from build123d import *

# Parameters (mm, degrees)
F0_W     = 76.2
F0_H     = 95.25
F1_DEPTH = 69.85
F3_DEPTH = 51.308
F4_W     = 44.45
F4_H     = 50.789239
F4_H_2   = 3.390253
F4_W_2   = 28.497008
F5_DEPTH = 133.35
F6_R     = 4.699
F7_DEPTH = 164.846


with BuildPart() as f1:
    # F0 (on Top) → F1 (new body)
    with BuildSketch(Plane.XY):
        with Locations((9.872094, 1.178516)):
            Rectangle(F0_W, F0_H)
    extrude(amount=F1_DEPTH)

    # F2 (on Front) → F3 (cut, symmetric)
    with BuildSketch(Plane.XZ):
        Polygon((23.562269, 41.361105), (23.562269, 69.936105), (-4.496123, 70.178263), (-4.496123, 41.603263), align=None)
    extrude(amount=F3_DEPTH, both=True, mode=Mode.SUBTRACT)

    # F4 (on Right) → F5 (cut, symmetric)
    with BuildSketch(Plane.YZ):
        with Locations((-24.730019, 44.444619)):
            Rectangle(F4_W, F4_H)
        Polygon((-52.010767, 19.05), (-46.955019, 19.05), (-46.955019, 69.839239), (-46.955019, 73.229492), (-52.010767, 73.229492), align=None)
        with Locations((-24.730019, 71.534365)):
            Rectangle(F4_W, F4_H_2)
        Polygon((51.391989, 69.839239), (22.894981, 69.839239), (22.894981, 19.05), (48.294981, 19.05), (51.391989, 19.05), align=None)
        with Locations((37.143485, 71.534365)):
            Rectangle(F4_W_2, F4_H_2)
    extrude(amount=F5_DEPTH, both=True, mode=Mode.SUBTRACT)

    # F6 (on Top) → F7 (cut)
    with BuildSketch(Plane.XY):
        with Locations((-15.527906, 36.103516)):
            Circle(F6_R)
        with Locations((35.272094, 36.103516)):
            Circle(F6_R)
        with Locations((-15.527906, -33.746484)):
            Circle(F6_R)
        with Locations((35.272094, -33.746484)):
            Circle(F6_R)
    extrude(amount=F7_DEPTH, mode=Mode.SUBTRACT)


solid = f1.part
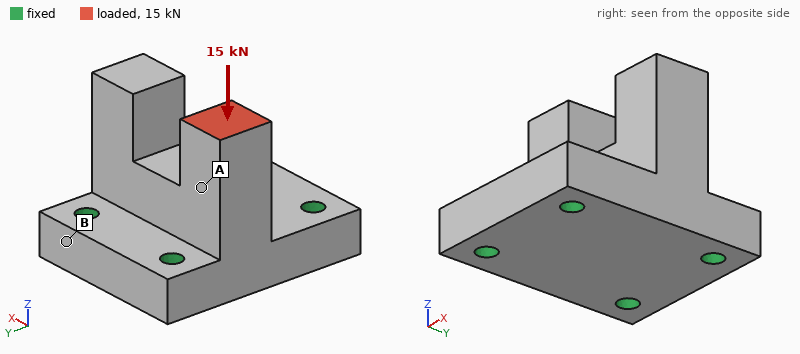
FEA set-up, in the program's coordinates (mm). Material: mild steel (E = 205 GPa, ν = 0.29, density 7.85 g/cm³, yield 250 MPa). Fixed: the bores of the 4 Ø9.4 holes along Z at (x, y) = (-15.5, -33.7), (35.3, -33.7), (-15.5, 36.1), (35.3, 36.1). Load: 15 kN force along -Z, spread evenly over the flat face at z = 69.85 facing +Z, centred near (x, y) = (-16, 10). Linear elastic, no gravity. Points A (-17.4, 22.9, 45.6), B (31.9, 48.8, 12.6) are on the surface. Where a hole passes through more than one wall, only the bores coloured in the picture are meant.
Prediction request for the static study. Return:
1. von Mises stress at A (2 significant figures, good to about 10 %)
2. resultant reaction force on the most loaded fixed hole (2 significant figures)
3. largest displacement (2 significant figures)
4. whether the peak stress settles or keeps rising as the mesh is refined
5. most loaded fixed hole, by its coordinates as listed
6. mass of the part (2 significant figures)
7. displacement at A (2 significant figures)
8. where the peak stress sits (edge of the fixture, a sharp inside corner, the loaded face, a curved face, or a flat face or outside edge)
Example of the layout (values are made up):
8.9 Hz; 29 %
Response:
23 MPa; 9.7 kN; 21 µm; keeps rising; (-15.5, 36.1); 1.7 kg; 11 µm; edge of the fixture
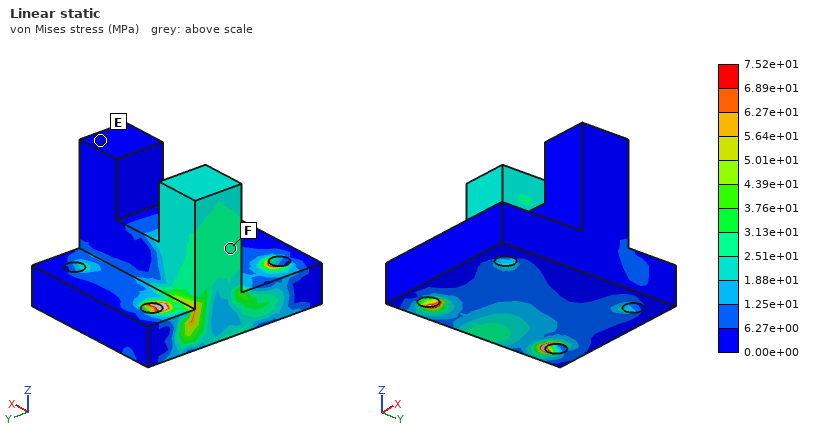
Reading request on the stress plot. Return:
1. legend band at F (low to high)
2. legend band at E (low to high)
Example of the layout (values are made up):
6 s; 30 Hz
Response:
2.51e+01 to 3.13e+01 MPa; 0.00e+00 to 6.27e+00 MPa
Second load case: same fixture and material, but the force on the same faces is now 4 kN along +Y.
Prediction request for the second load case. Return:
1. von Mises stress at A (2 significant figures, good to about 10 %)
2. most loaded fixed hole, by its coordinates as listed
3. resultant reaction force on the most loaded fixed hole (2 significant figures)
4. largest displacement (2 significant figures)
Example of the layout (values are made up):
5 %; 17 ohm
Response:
35 MPa; (-15.5, 36.1); 3.5 kN; 39 µm
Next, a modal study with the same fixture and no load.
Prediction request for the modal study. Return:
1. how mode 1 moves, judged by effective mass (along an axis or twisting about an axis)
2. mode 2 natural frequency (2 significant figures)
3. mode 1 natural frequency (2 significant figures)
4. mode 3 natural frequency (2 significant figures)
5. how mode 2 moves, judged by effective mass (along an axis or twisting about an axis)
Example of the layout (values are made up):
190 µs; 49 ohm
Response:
along Y; 6100 Hz; 5500 Hz; 6900 Hz; along X
